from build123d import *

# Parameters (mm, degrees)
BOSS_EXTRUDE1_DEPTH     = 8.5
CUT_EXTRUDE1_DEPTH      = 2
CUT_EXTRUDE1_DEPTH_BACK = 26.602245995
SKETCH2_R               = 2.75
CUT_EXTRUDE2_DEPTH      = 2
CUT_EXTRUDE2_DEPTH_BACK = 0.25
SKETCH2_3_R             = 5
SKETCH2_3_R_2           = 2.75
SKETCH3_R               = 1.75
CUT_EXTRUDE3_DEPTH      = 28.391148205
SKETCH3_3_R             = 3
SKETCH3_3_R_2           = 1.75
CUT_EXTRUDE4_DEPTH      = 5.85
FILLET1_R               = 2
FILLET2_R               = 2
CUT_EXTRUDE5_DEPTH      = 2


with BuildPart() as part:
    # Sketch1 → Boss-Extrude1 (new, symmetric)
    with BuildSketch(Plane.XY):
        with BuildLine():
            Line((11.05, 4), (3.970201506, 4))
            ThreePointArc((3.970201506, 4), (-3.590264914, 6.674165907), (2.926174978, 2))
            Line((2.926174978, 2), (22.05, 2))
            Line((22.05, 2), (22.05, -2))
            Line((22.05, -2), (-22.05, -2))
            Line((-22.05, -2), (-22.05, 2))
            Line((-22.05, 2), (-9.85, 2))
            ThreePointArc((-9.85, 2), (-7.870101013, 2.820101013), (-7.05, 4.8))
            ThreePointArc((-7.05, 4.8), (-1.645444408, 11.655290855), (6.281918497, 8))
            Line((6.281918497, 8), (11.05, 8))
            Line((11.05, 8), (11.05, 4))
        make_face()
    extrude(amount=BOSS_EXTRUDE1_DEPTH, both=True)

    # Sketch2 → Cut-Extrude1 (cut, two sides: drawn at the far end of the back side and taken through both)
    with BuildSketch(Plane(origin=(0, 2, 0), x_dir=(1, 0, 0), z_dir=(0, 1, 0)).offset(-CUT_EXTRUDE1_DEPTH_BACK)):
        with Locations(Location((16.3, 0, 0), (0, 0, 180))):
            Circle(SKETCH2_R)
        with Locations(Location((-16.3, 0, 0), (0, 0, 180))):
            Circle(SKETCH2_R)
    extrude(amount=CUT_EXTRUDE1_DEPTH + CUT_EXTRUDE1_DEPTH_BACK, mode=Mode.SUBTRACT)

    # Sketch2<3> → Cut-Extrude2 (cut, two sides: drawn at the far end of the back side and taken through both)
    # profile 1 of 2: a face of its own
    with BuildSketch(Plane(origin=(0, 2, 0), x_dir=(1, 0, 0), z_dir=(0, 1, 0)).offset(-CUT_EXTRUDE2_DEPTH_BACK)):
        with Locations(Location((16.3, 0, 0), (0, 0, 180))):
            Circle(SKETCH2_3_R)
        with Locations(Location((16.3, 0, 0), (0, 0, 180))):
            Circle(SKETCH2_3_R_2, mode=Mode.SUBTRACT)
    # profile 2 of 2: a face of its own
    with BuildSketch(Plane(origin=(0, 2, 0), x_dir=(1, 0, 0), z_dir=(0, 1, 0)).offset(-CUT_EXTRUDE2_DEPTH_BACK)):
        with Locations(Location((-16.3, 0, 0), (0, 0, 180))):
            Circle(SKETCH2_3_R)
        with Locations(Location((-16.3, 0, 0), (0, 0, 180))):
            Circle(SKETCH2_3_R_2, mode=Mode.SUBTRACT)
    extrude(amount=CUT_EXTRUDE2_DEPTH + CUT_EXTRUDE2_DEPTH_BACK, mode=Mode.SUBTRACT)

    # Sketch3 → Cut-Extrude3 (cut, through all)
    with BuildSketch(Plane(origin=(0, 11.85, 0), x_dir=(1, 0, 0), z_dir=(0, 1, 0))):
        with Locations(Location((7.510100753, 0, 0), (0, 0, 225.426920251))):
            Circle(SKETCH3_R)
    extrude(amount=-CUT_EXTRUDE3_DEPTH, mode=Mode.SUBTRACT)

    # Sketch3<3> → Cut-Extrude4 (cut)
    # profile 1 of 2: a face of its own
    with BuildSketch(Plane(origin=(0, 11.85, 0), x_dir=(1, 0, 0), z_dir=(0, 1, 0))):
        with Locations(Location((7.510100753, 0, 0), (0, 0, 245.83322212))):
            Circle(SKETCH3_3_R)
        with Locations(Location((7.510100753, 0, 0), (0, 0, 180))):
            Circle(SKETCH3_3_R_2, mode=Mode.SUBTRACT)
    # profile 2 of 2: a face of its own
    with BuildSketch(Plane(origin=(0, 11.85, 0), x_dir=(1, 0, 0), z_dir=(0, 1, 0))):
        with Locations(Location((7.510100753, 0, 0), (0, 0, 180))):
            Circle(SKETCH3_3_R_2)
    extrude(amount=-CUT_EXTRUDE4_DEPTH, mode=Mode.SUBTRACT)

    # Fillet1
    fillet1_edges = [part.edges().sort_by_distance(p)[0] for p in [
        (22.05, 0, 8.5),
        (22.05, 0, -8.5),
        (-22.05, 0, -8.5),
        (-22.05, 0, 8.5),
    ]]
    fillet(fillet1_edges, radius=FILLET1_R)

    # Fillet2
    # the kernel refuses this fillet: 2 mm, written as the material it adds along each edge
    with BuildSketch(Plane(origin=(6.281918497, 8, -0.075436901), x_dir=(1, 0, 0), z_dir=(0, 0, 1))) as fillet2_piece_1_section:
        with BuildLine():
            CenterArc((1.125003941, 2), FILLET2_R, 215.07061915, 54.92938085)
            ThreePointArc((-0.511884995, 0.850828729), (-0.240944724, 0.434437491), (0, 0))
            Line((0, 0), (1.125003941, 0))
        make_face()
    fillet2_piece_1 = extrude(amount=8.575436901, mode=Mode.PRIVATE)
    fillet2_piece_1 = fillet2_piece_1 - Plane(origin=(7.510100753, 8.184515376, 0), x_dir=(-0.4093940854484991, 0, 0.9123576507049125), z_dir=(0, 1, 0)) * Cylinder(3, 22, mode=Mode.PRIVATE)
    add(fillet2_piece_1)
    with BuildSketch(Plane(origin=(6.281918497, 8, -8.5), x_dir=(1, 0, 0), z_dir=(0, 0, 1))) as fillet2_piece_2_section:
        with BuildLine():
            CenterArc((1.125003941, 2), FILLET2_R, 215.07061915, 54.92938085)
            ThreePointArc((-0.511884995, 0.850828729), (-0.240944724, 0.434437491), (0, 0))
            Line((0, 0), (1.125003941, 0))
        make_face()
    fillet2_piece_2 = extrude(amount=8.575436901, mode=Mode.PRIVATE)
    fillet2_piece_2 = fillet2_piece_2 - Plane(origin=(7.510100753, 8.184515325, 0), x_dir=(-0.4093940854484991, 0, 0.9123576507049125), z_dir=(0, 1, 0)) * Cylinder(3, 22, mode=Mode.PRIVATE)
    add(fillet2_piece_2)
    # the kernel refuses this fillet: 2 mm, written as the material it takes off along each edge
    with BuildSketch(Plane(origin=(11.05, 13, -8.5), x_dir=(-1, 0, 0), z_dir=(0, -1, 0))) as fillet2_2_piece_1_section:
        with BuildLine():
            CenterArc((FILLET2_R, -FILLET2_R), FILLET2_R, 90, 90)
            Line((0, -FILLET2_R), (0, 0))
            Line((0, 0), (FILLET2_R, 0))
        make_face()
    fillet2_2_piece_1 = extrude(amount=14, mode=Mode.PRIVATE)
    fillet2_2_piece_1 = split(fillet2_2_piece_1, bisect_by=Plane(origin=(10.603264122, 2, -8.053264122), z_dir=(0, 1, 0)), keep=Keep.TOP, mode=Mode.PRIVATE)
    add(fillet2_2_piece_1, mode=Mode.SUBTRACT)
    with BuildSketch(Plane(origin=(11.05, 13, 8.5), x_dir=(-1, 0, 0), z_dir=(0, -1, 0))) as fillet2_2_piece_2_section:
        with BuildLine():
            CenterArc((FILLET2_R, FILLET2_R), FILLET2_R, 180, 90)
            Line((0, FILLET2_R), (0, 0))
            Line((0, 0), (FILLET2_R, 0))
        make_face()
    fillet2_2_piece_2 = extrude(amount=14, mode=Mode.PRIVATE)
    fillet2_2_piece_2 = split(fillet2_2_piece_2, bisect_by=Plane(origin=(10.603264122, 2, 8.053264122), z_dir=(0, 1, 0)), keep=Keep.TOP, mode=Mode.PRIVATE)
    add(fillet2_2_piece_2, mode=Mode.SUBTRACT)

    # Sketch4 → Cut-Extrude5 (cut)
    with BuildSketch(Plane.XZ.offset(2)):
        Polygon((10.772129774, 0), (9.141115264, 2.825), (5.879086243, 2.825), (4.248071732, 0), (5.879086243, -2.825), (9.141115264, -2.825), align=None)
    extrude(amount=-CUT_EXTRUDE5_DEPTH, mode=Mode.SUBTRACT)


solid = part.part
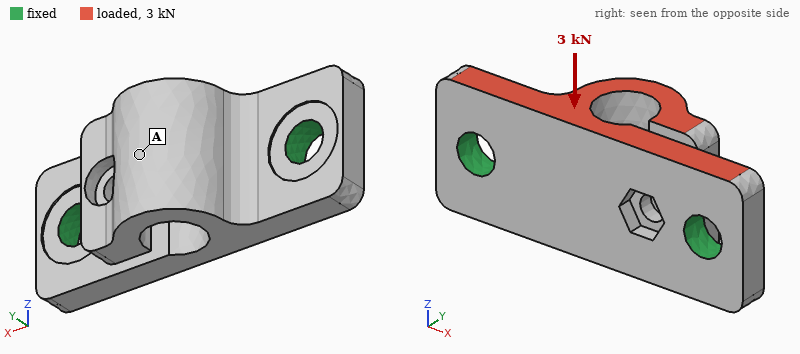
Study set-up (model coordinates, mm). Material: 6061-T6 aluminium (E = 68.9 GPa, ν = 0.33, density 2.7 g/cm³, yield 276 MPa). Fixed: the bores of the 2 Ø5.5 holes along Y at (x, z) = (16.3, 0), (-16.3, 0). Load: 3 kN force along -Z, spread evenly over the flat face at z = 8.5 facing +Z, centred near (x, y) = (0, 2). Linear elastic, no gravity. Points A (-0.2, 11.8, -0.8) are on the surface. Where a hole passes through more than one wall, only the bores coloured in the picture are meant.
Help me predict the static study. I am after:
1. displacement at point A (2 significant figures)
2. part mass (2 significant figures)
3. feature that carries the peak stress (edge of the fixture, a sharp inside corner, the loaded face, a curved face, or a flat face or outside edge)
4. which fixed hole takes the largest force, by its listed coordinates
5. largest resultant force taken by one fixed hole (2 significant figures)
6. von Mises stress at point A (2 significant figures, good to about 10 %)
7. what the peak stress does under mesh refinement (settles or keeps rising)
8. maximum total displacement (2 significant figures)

0.075 mm
11 g
edge of the fixture
(-16.3, 0)
1.6 kN
32 MPa
keeps rising
0.15 mm
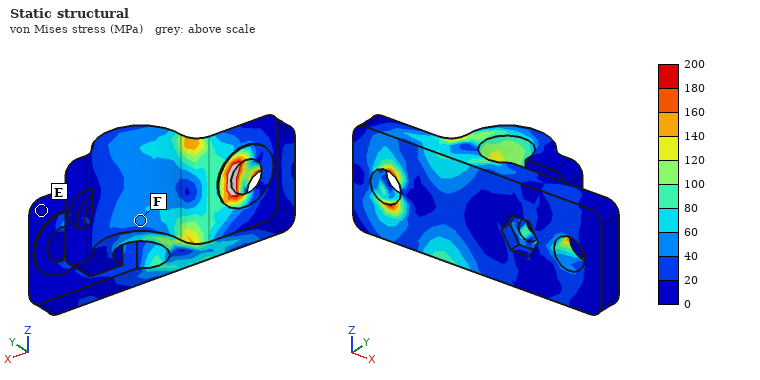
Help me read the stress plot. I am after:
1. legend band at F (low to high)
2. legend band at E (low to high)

40 to 60 MPa
0 to 20 MPa
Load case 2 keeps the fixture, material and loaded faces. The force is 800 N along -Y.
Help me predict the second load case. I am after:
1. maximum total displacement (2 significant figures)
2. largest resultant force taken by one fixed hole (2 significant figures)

0.16 mm
420 N
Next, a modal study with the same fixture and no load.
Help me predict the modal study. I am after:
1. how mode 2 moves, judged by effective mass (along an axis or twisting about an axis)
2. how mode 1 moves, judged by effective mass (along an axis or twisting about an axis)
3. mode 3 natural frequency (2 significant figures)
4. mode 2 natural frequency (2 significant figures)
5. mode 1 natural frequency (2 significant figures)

along Z
along Y
11 kHz
7800 Hz
4700 Hz
